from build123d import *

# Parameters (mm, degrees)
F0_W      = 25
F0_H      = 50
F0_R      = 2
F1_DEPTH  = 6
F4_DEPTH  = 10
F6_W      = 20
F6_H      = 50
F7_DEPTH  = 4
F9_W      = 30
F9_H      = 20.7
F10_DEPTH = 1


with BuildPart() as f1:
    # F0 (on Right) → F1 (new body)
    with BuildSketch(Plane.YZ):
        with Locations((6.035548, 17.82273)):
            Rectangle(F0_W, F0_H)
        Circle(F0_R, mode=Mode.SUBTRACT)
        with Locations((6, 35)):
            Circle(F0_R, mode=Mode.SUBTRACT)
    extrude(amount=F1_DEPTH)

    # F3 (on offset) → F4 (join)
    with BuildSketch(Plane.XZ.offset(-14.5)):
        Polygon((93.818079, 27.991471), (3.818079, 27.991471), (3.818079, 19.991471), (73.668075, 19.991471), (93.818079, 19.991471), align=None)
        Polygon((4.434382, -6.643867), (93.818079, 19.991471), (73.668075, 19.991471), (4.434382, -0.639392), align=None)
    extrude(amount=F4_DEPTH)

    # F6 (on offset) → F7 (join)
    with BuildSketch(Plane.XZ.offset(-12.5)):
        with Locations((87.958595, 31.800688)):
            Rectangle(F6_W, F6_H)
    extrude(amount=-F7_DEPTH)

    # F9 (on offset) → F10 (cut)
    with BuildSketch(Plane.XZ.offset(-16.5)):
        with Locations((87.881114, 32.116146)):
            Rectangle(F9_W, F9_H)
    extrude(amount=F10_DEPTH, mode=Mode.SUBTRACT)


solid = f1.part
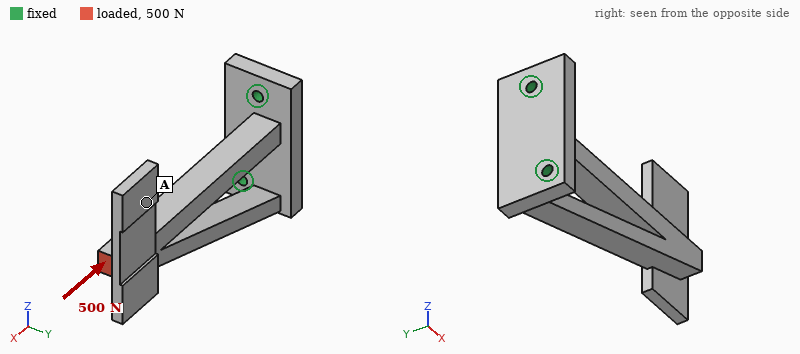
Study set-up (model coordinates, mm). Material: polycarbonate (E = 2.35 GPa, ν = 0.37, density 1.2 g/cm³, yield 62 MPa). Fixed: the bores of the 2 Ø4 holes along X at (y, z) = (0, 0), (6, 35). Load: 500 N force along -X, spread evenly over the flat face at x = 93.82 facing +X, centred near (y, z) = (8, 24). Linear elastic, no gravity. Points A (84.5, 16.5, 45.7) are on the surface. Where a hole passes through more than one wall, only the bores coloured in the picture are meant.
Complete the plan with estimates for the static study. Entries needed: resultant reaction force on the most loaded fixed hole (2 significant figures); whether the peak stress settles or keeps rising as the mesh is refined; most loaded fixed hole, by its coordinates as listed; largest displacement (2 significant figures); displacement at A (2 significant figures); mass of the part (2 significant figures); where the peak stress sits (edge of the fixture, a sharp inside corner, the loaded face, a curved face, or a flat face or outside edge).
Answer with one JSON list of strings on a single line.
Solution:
["380 N", "keeps rising", "(6, 35)", "1.3 mm", "0.93 mm", "27 g", "edge of the fixture"]
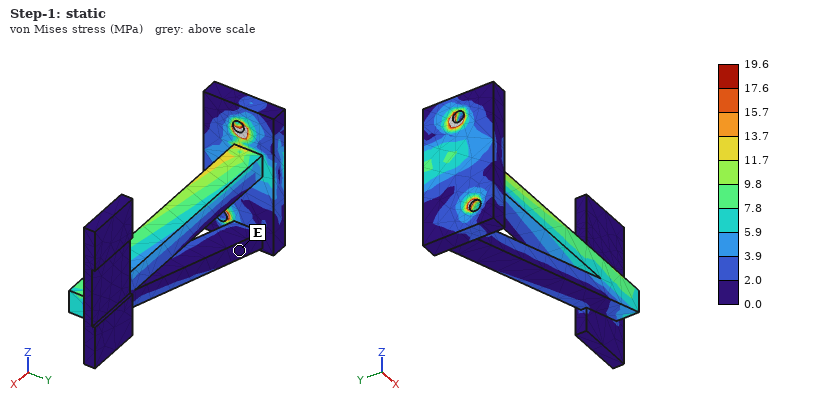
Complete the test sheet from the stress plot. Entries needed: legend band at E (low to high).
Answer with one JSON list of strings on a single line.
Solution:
["0.0 to 2.0 MPa"]
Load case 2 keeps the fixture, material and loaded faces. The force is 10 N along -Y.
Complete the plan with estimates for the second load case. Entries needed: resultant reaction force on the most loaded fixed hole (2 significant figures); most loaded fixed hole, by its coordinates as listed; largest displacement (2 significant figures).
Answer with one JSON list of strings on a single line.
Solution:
["7.8 N", "(6, 35)", "1.4 mm"]
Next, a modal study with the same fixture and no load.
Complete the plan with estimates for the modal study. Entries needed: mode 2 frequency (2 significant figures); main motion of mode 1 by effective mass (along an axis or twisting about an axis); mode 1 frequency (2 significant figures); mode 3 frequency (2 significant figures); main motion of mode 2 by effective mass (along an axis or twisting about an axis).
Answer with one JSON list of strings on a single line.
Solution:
["450 Hz", "along Y", "170 Hz", "490 Hz", "along Z"]
